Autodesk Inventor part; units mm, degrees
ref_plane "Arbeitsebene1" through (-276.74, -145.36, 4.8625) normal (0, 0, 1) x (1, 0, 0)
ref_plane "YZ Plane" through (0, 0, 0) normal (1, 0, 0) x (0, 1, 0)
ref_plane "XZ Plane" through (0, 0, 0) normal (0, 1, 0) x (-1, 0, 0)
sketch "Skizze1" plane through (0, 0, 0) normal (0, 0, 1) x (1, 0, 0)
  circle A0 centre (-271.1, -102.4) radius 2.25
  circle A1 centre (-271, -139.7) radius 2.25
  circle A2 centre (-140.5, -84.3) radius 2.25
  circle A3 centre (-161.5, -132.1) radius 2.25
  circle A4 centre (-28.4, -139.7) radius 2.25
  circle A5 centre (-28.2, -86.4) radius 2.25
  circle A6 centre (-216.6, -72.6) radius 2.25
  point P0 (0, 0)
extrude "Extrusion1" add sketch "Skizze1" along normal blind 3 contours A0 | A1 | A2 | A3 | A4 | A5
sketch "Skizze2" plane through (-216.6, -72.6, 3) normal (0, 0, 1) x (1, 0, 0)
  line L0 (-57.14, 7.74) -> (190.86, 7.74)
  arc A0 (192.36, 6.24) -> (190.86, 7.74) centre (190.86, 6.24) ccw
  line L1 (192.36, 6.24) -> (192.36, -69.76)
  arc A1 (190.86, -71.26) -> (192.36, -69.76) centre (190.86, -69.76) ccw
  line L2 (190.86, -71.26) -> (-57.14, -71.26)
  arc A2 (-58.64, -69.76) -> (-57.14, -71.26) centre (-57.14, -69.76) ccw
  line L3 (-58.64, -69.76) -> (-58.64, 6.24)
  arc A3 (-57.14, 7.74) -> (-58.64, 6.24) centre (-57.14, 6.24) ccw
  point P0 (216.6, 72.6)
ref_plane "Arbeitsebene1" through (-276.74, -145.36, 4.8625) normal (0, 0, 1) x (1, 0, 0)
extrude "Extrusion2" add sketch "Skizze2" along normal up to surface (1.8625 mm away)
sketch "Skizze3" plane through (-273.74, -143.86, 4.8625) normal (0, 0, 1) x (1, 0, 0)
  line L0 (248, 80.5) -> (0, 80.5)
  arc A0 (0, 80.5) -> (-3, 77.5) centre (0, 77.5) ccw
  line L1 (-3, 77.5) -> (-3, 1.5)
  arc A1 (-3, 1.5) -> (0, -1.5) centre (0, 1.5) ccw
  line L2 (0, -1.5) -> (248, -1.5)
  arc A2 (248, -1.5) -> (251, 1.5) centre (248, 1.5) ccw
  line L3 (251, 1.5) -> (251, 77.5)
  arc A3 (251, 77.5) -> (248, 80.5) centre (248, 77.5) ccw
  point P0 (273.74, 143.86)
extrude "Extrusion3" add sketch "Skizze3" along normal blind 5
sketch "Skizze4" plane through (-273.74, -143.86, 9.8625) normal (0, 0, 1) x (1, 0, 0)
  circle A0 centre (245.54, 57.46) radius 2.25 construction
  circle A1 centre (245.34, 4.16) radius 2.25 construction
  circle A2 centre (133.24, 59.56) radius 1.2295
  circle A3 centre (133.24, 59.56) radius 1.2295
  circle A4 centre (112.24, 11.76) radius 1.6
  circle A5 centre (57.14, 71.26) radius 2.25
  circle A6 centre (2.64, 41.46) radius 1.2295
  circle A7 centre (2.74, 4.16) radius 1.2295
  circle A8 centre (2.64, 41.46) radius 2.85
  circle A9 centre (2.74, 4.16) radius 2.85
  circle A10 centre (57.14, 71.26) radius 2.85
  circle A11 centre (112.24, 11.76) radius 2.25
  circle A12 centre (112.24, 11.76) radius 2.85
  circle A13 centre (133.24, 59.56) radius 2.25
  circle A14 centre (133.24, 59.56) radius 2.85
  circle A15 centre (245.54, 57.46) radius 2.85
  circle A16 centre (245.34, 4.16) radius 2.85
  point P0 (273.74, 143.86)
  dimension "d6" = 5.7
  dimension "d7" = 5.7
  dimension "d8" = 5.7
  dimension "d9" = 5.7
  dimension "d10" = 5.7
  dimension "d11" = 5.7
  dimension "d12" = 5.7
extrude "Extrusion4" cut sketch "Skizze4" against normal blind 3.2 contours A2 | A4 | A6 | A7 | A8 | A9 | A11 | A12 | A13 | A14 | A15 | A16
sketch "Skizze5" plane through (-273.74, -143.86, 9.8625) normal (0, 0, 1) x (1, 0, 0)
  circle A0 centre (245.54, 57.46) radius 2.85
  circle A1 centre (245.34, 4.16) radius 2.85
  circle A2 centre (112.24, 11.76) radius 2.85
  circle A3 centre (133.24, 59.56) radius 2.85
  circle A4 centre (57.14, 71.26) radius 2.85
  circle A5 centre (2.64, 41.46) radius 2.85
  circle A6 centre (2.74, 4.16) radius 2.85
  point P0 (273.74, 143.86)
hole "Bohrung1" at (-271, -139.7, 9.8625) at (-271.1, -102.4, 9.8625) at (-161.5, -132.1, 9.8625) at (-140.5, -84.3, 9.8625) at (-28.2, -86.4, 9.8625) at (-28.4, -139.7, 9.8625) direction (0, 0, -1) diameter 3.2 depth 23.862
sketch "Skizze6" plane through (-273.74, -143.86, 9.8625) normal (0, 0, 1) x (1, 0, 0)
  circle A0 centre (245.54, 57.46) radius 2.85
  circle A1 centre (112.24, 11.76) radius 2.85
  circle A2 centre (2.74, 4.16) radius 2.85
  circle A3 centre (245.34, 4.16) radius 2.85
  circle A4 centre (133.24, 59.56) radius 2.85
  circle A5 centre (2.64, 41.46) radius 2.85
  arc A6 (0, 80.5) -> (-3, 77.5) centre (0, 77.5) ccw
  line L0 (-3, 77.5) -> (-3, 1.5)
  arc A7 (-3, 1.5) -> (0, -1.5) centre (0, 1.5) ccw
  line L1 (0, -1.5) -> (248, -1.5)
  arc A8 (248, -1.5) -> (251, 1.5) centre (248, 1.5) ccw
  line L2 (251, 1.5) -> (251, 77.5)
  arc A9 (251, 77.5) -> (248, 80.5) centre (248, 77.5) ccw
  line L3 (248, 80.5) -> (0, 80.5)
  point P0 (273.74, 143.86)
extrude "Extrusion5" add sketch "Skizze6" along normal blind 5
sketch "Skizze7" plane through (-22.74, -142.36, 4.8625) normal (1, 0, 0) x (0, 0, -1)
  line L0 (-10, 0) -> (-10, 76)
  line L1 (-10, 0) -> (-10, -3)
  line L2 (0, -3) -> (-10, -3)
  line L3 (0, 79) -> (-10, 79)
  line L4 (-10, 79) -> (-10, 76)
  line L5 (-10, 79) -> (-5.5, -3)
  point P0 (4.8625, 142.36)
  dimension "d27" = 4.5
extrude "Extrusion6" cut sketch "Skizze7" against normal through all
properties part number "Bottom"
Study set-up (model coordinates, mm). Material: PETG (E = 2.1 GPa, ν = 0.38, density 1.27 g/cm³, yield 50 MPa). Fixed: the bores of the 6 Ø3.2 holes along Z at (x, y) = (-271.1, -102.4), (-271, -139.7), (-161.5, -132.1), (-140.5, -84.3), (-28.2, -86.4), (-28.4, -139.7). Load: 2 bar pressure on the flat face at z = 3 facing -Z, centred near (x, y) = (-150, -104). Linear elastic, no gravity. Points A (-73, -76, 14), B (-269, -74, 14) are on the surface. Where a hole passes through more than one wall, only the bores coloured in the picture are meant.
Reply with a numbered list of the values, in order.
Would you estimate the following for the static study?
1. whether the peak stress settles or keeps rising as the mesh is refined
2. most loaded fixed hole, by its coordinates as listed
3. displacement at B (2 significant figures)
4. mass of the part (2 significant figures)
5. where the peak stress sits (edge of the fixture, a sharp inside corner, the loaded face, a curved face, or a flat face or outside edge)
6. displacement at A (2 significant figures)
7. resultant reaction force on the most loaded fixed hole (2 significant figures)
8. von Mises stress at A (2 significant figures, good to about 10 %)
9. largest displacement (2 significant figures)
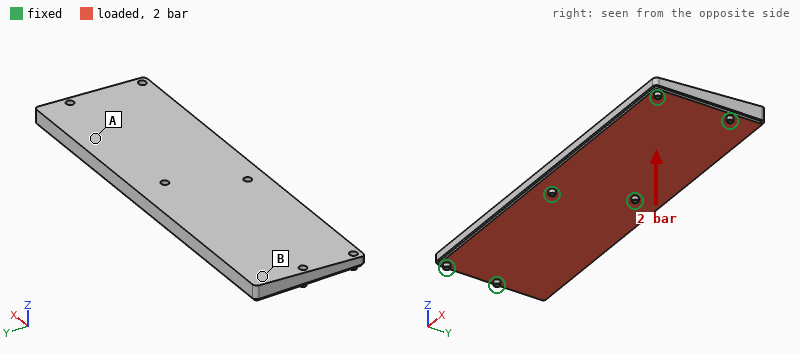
1. keeps rising
2. (-140.5, -84.3)
3. 0.78 mm
4. 250 g
5. edge of the fixture
6. 0.81 mm
7. 1.4 kN
8. 9.9 MPa
9. 1.9 mm
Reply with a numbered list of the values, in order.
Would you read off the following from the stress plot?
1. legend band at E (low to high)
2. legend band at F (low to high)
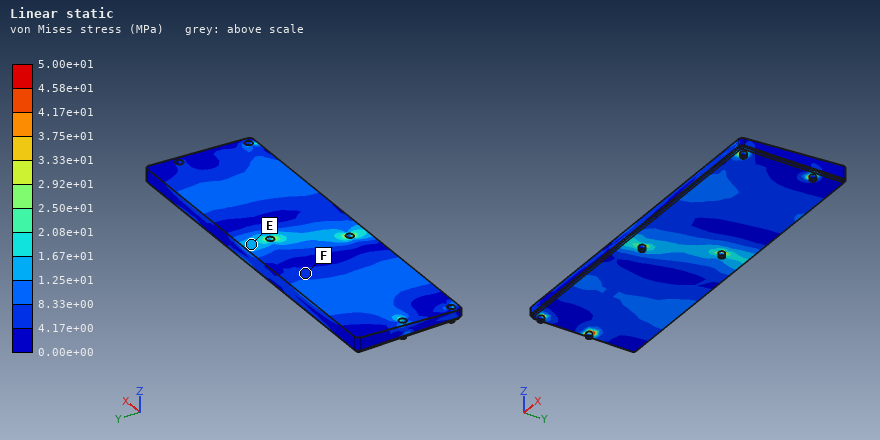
1. 1.25e+01 to 1.67e+01 MPa
2. 4.17e+00 to 8.33e+00 MPa
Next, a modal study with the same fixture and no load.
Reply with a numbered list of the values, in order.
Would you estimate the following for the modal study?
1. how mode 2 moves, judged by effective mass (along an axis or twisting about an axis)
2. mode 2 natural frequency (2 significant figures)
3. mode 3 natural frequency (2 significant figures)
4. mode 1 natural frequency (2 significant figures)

1. along Z
2. 620 Hz
3. 810 Hz
4. 470 Hz
